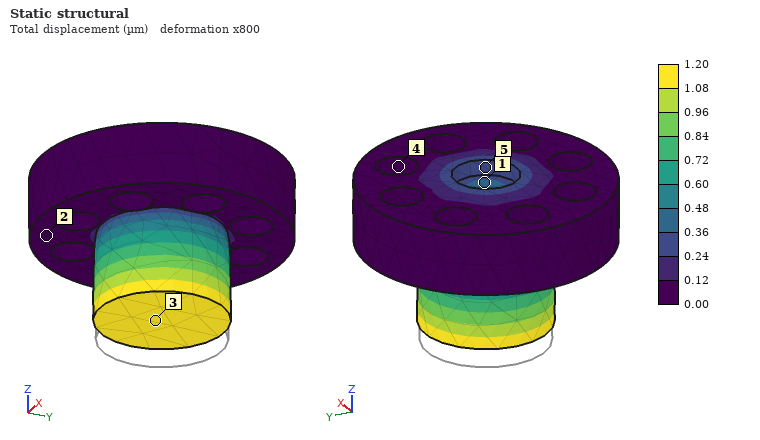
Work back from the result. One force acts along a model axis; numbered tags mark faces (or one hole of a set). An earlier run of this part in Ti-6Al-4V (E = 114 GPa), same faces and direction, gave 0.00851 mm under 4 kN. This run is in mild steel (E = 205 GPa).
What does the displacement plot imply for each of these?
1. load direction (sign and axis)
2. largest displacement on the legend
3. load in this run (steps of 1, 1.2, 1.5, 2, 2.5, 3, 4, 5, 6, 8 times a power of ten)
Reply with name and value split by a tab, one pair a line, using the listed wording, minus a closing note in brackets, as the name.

load direction	+Z
largest displacement on the legend	1.20 µm
load in this run	1 kN
